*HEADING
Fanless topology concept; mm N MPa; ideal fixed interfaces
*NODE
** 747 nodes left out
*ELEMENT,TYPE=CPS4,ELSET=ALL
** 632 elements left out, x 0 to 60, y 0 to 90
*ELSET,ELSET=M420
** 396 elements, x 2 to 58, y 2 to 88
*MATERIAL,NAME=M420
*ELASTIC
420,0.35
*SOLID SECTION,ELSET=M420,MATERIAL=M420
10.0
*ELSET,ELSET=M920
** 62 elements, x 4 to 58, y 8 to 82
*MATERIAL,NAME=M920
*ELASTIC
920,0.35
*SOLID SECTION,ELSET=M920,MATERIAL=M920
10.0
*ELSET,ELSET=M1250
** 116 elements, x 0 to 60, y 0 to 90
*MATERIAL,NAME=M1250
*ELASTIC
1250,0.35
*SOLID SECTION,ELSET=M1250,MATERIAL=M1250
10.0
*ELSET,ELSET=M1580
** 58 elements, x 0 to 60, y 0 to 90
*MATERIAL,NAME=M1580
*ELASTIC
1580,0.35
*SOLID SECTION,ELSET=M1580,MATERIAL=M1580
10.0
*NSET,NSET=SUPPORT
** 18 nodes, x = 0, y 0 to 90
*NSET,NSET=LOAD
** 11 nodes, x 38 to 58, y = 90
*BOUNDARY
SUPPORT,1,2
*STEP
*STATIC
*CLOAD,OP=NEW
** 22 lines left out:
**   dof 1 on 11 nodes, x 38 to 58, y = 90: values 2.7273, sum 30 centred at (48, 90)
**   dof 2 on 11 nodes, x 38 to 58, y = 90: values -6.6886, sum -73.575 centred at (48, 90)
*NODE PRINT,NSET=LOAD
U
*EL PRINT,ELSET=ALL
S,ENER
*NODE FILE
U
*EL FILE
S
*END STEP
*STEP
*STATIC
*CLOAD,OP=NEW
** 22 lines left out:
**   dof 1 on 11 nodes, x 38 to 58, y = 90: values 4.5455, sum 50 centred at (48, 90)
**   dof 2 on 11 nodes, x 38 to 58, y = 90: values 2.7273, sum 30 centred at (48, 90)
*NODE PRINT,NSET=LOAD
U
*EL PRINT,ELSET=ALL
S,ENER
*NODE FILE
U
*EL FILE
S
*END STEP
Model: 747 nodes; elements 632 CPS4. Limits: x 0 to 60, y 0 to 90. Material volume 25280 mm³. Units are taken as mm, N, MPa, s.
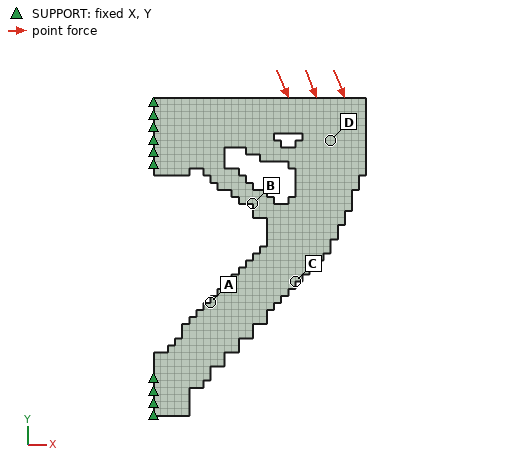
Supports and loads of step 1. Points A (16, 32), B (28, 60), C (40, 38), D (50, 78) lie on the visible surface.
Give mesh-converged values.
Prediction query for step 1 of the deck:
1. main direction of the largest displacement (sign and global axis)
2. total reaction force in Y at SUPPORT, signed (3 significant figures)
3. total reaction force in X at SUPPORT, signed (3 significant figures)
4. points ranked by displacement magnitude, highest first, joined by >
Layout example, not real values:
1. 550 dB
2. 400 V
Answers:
1. -Y
2. 73.6 N
3. -30.0 N
4. D > C > B > A
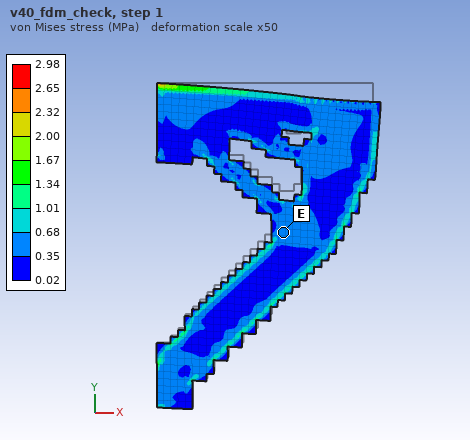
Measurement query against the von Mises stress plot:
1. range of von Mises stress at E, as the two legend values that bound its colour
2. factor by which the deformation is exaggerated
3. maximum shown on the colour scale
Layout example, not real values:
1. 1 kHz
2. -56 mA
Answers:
1. 0.35 to 0.68 MPa
2. 50
3. 2.98 MPa
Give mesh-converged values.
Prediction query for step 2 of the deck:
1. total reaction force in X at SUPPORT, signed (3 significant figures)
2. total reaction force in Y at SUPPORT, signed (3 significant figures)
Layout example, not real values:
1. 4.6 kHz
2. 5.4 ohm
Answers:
1. -50.0 N
2. -30.0 N
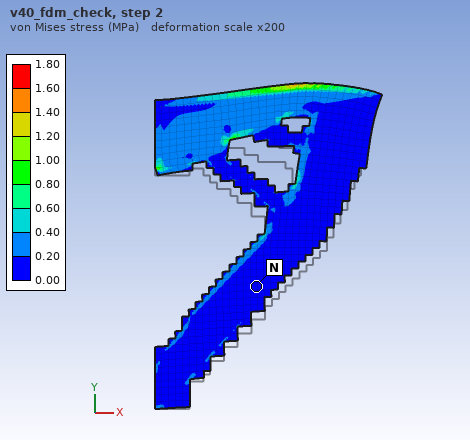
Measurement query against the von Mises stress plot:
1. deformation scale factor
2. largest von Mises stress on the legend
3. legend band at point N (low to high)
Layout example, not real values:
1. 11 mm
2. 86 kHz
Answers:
1. 200
2. 1.80 MPa
3. 0.00 to 0.20 MPa
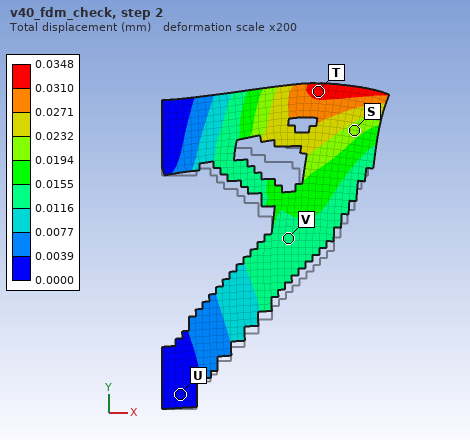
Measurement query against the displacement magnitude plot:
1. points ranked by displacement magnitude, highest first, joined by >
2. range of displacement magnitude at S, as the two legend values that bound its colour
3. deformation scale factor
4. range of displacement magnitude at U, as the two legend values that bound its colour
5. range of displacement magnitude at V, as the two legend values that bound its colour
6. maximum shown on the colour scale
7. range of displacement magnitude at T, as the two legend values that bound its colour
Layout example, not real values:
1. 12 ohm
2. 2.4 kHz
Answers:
1. T > S > V > U
2. 0.0194 to 0.0232 mm
3. 200
4. 0.0000 to 0.0039 mm
5. 0.0116 to 0.0155 mm
6. 0.0348 mm
7. 0.0310 to 0.0348 mm
